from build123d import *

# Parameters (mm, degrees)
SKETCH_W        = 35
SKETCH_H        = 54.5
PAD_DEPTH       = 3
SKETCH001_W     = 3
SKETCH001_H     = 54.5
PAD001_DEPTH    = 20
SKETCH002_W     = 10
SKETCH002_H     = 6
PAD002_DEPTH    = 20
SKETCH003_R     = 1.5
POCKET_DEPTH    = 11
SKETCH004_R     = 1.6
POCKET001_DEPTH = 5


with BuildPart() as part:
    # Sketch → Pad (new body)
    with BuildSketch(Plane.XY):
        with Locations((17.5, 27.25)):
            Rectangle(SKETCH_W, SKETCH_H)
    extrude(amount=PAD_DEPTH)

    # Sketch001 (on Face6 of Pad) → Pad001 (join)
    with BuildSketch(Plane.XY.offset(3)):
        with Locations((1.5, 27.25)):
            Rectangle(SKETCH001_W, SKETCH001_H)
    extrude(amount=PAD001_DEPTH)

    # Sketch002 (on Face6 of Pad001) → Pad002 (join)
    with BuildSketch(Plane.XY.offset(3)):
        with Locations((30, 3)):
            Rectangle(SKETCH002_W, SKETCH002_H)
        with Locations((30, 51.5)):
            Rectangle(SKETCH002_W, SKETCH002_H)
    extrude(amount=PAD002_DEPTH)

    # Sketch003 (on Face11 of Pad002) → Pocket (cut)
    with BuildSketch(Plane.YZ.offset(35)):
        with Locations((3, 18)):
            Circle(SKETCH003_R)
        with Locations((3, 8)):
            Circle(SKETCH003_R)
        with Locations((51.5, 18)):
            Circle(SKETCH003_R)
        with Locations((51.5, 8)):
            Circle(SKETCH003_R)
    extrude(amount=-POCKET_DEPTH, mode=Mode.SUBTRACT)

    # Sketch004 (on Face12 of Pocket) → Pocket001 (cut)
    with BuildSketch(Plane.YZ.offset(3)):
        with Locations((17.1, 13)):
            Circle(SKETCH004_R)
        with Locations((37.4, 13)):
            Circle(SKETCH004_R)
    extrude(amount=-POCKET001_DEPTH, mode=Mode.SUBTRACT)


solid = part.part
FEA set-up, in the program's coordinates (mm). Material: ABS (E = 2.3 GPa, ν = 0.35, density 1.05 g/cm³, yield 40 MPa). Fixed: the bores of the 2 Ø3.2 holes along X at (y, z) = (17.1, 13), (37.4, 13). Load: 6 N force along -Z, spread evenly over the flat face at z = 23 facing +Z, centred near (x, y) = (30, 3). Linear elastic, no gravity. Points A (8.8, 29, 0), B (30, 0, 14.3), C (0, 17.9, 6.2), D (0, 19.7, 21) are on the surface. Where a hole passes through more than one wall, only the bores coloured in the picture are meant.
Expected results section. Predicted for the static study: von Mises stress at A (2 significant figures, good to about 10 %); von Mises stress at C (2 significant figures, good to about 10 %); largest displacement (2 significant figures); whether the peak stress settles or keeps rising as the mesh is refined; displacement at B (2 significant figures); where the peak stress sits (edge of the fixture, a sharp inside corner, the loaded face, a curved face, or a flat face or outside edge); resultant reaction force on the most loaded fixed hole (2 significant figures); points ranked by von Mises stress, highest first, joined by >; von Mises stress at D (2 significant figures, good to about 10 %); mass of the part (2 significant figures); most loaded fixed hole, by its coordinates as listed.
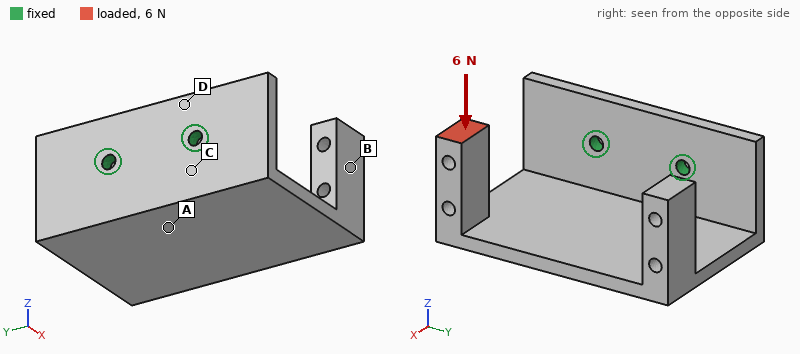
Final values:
1.5 MPa
2.5 MPa
0.77 mm
keeps rising
0.59 mm
edge of the fixture
9.4 N
C > A > D > B
0.76 MPa
12 g
(17.1, 13)
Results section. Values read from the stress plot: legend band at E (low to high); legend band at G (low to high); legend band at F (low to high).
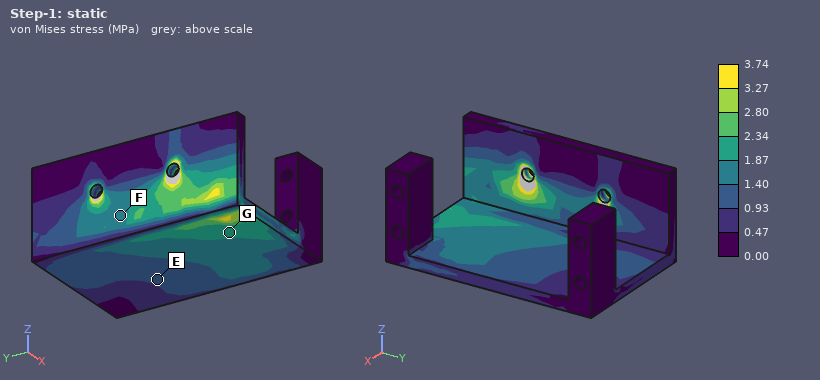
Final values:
0.93 to 1.40 MPa
1.87 to 2.34 MPa
1.40 to 1.87 MPa
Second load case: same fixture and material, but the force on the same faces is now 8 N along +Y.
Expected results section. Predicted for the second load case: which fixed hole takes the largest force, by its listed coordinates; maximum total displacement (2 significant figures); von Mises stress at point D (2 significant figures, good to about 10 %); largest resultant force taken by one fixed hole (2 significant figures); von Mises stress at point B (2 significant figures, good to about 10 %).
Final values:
(17.1, 13)
0.81 mm
0.53 MPa
11 N
1.3 MPa
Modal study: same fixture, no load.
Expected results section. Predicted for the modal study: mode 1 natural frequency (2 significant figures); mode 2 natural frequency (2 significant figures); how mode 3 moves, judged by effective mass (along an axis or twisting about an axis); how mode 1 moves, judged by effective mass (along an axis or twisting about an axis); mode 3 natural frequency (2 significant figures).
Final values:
290 Hz
430 Hz
along Y
along Z
660 Hz
